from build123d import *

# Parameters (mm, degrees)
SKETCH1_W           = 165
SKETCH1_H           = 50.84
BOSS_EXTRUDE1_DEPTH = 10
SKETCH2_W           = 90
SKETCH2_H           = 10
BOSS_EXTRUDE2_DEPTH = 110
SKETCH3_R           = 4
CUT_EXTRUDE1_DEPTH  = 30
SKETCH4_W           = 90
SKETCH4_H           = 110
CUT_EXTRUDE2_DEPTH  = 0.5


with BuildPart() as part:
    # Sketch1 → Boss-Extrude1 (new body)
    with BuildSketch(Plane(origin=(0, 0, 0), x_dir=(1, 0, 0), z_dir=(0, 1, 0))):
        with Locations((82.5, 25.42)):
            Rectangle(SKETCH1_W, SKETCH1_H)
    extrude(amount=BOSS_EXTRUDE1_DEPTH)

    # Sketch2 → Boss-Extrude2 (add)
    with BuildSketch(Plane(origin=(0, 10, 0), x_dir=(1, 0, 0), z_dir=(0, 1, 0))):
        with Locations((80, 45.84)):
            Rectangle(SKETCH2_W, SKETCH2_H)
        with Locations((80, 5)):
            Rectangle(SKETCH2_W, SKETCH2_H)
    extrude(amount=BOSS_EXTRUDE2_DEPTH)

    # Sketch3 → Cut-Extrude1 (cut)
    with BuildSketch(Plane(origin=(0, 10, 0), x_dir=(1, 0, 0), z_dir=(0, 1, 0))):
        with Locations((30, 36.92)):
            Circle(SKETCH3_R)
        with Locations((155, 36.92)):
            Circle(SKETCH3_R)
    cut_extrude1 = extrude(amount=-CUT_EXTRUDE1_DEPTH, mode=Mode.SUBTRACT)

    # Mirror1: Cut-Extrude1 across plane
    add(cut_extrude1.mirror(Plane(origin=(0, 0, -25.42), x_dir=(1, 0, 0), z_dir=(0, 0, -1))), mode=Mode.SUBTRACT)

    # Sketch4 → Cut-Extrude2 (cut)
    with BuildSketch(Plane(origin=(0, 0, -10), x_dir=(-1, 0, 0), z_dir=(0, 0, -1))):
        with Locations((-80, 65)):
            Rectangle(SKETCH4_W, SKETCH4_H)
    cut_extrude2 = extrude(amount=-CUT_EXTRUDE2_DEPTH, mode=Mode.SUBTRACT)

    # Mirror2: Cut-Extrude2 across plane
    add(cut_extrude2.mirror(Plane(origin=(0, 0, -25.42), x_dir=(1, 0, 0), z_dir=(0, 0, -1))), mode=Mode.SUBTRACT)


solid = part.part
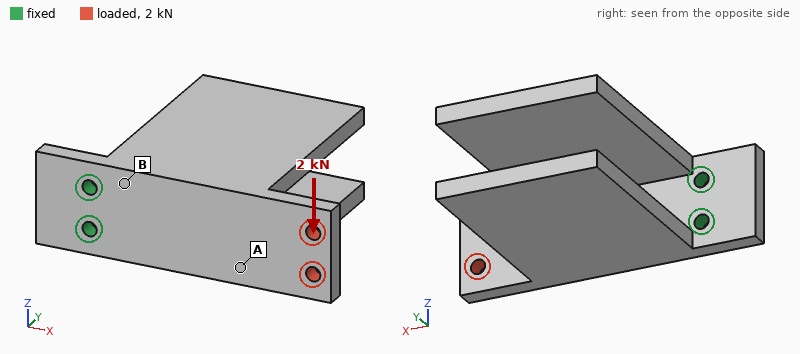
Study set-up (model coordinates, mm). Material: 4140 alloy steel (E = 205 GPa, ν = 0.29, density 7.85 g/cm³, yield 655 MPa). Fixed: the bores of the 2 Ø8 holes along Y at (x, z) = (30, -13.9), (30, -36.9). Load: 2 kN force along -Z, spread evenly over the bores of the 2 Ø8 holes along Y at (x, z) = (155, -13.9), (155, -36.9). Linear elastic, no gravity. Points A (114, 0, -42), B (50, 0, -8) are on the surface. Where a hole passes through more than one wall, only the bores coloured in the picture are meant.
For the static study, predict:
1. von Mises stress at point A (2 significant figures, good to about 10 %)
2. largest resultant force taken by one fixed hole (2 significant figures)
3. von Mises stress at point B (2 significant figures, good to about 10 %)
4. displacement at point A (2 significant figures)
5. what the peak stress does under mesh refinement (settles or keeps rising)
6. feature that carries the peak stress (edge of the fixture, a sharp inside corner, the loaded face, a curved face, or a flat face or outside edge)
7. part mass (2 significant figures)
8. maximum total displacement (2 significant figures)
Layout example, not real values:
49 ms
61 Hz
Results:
10 MPa
8.8 kN
30 MPa
34 µm
keeps rising
edge of the fixture
2.1 kg
65 µm
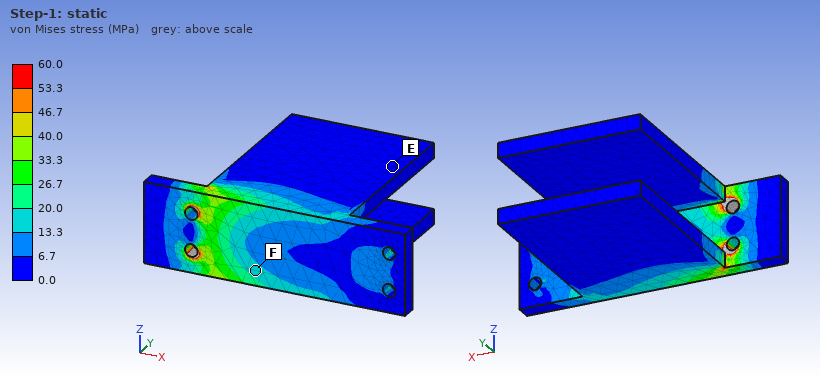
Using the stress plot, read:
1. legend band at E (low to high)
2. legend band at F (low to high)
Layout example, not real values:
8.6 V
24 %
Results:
0.0 to 6.7 MPa
13.3 to 20.0 MPa
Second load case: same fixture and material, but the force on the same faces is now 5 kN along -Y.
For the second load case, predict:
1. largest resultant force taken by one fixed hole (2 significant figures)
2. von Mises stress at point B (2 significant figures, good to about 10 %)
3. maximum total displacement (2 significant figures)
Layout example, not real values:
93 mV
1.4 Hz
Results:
3.3 kN
180 MPa
1.3 mm
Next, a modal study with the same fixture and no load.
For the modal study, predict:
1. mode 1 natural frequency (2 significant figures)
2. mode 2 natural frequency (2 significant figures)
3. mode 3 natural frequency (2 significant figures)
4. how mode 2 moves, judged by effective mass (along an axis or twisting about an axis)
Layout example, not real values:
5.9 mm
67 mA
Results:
360 Hz
380 Hz
520 Hz
along Z
